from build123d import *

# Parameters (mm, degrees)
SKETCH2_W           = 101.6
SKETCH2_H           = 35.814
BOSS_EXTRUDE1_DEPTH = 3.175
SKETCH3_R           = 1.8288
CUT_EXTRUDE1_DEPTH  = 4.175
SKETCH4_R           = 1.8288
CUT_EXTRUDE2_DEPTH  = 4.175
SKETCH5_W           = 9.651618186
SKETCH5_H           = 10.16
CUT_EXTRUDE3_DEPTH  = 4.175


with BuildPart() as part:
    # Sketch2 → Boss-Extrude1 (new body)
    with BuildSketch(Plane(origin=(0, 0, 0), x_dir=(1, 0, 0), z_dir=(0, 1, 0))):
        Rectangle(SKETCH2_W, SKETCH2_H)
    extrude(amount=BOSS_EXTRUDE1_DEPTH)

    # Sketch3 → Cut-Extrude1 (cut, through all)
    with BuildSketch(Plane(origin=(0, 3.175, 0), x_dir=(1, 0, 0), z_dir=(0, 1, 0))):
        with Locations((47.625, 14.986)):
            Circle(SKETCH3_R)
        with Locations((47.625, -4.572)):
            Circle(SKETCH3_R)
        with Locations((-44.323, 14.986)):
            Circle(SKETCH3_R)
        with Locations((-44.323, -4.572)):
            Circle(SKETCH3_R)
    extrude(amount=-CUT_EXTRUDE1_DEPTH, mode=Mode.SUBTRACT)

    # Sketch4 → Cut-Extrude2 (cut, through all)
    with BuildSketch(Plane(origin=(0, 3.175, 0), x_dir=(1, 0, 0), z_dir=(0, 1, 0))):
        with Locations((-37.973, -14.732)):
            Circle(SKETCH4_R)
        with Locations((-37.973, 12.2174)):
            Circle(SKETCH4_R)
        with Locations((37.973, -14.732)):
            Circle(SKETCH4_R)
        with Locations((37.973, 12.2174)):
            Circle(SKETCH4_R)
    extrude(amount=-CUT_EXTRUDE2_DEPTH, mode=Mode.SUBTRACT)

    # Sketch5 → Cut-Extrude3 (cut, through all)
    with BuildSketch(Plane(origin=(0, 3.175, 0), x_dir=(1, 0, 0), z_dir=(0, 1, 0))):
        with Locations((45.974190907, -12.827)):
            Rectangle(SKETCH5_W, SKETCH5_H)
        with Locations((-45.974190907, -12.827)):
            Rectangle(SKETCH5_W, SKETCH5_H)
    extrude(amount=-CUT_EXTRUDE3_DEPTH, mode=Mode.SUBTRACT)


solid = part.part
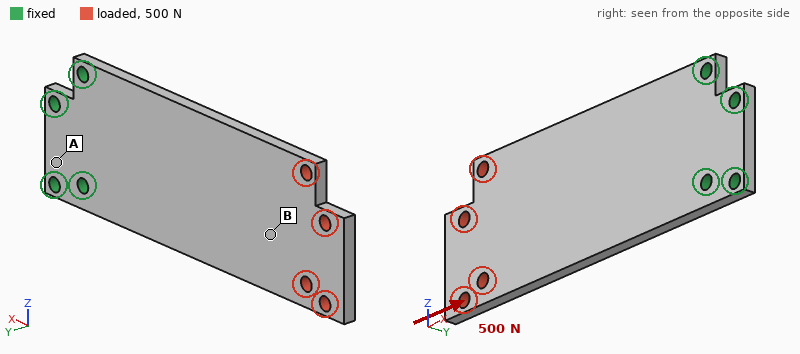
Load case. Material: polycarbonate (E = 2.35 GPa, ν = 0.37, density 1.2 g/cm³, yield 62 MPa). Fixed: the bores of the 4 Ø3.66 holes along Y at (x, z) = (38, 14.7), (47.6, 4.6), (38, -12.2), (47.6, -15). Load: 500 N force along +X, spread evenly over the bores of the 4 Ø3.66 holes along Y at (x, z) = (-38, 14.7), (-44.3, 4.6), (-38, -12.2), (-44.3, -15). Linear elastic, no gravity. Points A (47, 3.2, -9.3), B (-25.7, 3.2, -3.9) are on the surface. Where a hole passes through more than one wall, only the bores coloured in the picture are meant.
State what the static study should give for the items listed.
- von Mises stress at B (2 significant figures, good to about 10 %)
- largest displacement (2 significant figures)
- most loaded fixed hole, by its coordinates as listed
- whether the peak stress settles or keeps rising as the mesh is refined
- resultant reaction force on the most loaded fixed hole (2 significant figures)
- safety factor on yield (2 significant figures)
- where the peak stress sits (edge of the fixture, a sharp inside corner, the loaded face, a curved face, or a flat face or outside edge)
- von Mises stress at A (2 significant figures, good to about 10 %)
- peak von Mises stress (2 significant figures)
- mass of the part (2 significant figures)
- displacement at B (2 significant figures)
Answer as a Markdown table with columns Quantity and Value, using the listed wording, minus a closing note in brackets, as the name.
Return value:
| Quantity | Value |
|---|---|
| von Mises stress at B | 4.2 MPa |
| largest displacement | 0.28 mm |
| most loaded fixed hole, by its coordinates as listed | (38, -12.2) |
| whether the peak stress settles or keeps rising as the mesh is refined | settles |
| resultant reaction force on the most loaded fixed hole | 230 N |
| safety factor on yield | 3.3 |
| where the peak stress sits | the loaded face |
| von Mises stress at A | 1.5 MPa |
| peak von Mises stress | 19 MPa |
| mass of the part | 13 g |
| displacement at B | 0.15 mm |
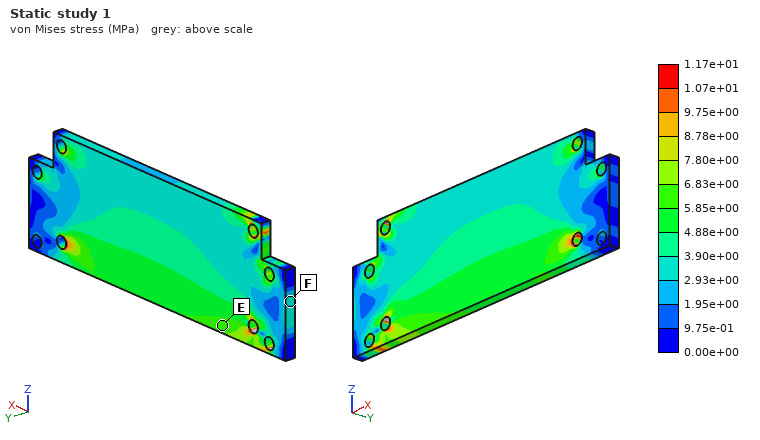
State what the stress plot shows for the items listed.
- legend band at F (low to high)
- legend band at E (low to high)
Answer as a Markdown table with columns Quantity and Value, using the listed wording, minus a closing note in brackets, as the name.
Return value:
| Quantity | Value |
|---|---|
| legend band at F | 2.93e+00 to 3.90e+00 MPa |
| legend band at E | 5.85e+00 to 6.83e+00 MPa |
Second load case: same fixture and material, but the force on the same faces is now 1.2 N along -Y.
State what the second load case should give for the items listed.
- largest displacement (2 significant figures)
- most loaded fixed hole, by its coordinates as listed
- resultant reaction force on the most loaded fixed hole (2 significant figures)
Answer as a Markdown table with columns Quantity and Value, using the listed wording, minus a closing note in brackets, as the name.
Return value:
| Quantity | Value |
|---|---|
| largest displacement | 1.0 mm |
| most loaded fixed hole, by its coordinates as listed | (38, -12.2) |
| resultant reaction force on the most loaded fixed hole | 2.8 N |
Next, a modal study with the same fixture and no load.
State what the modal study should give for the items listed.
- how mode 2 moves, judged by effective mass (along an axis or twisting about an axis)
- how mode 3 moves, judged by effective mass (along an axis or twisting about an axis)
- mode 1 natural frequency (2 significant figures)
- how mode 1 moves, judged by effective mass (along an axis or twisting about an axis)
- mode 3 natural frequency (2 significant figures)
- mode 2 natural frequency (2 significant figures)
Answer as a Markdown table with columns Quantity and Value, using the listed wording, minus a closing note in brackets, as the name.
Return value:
| Quantity | Value |
|---|---|
| how mode 2 moves, judged by effective mass | twisting about X |
| how mode 3 moves, judged by effective mass | along Y |
| mode 1 natural frequency | 99 Hz |
| how mode 1 moves, judged by effective mass | along Y |
| mode 3 natural frequency | 610 Hz |
| mode 2 natural frequency | 500 Hz |
